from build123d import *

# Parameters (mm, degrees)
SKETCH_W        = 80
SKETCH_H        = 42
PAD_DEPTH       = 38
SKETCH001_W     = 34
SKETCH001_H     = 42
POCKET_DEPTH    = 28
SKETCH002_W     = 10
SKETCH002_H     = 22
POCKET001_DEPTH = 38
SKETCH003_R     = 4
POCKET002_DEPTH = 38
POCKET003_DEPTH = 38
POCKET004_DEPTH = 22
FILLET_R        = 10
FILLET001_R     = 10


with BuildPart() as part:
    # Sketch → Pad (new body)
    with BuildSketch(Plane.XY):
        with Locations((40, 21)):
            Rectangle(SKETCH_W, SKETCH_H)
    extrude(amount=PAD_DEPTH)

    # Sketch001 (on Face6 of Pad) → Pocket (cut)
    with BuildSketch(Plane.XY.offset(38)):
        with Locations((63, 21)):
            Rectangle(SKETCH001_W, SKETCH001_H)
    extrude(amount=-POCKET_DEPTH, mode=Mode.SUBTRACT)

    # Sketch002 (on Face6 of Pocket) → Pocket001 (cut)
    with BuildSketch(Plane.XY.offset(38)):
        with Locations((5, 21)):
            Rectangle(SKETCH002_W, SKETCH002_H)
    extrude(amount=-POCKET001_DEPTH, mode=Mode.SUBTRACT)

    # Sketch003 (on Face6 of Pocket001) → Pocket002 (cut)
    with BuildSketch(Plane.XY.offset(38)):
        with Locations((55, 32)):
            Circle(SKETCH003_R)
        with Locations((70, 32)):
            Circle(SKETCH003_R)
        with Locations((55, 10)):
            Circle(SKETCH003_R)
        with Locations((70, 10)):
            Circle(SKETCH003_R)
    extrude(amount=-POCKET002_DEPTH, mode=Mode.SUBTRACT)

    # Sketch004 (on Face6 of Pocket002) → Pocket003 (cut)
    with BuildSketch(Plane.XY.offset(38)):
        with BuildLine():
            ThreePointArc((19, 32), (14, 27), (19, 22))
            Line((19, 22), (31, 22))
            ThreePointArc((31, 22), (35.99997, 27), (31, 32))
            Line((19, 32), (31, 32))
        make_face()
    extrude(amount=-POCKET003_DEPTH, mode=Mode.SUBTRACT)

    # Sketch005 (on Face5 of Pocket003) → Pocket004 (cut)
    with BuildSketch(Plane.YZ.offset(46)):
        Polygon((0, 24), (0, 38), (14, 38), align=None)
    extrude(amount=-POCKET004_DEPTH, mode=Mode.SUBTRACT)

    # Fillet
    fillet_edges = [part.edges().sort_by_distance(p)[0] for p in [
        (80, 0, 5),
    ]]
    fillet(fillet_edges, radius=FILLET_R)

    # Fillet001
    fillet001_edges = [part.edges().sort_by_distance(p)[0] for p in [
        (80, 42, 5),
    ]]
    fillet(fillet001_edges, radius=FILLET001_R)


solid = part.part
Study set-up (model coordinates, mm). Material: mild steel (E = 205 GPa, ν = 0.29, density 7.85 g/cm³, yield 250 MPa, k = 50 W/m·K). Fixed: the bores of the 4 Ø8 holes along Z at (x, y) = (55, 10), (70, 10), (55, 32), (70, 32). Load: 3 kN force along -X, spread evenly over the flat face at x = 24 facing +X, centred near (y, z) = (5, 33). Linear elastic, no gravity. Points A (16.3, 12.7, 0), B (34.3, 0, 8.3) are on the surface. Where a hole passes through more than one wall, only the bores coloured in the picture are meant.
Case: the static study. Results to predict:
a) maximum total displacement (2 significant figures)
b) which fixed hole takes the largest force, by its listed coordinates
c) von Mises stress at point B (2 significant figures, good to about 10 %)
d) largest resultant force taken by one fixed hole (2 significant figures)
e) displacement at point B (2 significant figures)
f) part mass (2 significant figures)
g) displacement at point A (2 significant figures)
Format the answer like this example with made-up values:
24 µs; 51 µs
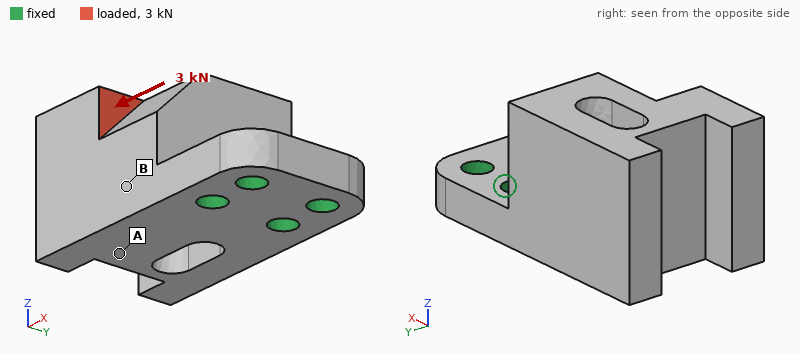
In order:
91 µm; (55, 10); 25 MPa; 3.0 kN; 20 µm; 530 g; 47 µm
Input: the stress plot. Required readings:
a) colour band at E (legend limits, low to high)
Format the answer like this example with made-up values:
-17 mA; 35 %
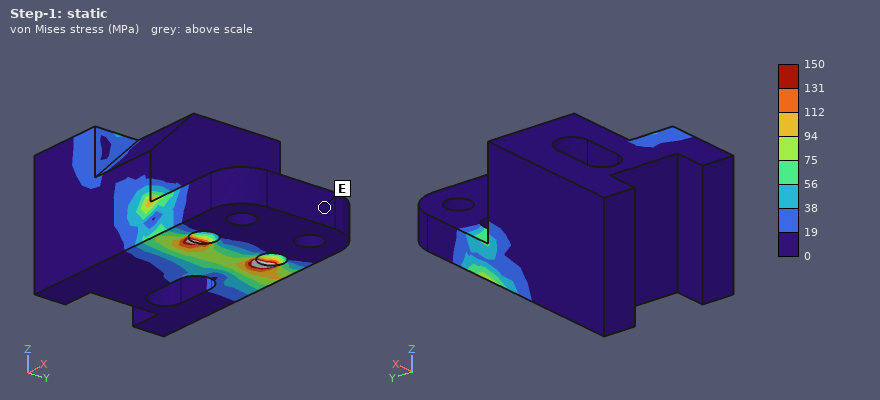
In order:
0 to 19 MPa
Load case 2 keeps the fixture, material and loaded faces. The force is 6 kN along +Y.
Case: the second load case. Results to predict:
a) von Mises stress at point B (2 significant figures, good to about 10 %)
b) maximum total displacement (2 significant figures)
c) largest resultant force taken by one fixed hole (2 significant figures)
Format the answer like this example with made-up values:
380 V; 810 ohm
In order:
20 MPa; 44 µm; 8.8 kN
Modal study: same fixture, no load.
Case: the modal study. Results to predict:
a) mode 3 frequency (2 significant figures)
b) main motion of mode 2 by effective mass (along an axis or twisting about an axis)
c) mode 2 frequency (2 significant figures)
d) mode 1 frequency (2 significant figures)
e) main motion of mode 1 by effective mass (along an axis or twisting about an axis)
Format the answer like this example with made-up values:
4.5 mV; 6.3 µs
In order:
6300 Hz; along Y; 4700 Hz; 1800 Hz; along Z
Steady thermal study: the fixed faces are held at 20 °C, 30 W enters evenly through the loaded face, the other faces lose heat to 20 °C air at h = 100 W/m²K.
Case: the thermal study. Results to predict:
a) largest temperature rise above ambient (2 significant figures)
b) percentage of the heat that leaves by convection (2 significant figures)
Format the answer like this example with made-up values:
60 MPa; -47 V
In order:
65 K; 55 %
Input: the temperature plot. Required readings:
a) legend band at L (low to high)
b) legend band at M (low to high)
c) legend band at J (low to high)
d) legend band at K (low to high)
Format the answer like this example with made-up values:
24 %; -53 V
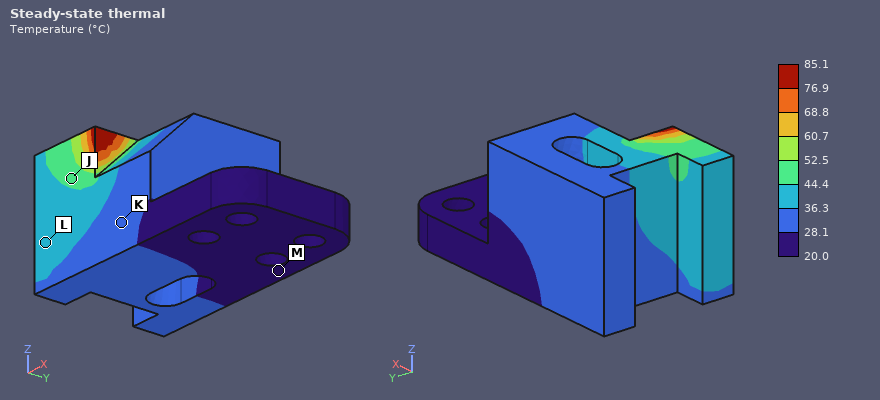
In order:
36.3 to 44.4 °C; 20.0 to 28.1 °C; 44.4 to 52.5 °C; 28.1 to 36.3 °C
